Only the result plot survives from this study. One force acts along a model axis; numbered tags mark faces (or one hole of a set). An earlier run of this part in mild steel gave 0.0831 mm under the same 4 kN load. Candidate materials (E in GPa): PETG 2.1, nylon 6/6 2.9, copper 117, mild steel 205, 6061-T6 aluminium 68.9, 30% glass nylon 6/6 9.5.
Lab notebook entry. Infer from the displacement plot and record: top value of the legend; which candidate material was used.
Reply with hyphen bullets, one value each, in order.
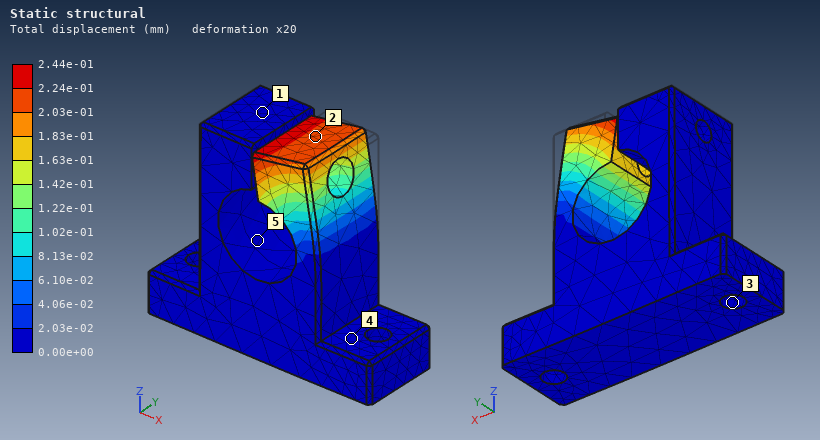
- 2.44e-01 mm
- 6061-T6 aluminium
